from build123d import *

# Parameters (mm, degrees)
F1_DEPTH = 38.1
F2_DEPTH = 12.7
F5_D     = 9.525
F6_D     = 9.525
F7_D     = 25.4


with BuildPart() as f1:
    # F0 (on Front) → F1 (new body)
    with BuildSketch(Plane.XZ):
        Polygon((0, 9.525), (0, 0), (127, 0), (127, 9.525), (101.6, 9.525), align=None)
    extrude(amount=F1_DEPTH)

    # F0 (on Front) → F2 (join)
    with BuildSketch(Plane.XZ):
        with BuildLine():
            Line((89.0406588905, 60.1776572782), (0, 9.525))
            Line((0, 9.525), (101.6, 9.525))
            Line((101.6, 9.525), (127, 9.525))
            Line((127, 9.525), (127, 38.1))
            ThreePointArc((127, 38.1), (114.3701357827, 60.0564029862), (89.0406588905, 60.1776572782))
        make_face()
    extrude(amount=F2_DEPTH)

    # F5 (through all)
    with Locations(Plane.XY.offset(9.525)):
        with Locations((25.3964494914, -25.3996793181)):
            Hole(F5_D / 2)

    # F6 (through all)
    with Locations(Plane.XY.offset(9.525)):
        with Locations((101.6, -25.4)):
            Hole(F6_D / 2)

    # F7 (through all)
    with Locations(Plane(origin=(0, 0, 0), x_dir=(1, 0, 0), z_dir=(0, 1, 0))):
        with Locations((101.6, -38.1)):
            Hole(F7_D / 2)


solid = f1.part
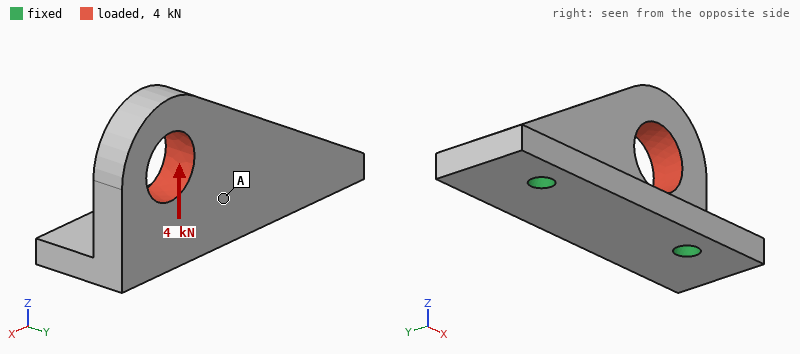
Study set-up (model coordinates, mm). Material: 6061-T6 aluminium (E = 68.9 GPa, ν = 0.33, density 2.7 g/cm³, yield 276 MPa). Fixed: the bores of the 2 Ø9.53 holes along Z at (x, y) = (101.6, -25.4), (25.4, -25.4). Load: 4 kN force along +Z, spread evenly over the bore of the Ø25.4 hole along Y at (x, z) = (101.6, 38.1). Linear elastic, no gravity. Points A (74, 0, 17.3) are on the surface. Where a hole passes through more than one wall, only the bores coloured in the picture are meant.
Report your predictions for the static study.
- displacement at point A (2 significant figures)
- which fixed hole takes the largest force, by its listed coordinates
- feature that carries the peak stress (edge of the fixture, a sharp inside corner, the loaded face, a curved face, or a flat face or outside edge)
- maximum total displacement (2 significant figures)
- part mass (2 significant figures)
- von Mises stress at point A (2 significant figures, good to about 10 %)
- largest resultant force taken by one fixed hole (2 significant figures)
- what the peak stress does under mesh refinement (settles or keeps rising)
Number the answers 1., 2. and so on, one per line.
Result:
1. 0.044 mm
2. (101.6, -25.4)
3. edge of the fixture
4. 0.13 mm
5. 250 g
6. 9.6 MPa
7. 3.9 kN
8. keeps rising
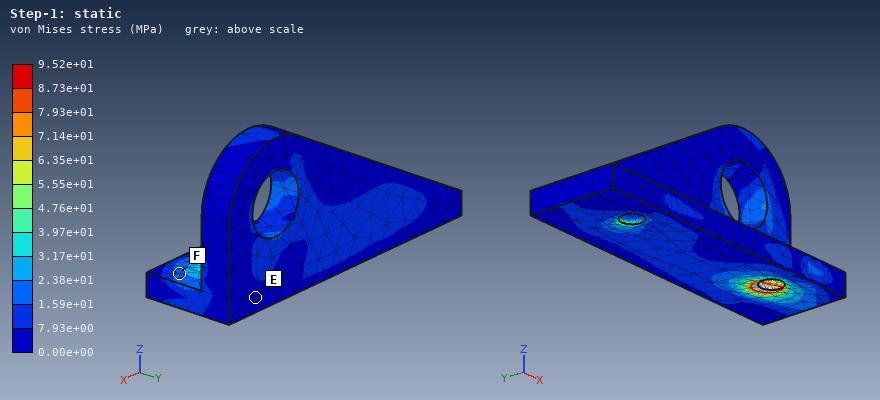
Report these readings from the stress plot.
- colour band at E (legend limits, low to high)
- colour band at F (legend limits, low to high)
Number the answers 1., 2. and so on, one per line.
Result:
1. 0.00e+00 to 7.93e+00 MPa
2. 1.59e+01 to 2.38e+01 MPa
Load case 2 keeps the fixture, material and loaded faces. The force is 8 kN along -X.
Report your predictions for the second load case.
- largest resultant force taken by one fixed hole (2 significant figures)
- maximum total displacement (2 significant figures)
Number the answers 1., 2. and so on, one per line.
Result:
1. 5.5 kN
2. 94 µm
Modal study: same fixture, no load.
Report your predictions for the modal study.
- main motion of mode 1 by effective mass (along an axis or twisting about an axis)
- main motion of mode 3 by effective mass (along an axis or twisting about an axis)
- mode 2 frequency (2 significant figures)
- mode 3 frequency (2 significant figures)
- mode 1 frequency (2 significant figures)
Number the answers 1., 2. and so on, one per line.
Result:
1. along Y
2. along Z
3. 4900 Hz
4. 6200 Hz
5. 2100 Hz
